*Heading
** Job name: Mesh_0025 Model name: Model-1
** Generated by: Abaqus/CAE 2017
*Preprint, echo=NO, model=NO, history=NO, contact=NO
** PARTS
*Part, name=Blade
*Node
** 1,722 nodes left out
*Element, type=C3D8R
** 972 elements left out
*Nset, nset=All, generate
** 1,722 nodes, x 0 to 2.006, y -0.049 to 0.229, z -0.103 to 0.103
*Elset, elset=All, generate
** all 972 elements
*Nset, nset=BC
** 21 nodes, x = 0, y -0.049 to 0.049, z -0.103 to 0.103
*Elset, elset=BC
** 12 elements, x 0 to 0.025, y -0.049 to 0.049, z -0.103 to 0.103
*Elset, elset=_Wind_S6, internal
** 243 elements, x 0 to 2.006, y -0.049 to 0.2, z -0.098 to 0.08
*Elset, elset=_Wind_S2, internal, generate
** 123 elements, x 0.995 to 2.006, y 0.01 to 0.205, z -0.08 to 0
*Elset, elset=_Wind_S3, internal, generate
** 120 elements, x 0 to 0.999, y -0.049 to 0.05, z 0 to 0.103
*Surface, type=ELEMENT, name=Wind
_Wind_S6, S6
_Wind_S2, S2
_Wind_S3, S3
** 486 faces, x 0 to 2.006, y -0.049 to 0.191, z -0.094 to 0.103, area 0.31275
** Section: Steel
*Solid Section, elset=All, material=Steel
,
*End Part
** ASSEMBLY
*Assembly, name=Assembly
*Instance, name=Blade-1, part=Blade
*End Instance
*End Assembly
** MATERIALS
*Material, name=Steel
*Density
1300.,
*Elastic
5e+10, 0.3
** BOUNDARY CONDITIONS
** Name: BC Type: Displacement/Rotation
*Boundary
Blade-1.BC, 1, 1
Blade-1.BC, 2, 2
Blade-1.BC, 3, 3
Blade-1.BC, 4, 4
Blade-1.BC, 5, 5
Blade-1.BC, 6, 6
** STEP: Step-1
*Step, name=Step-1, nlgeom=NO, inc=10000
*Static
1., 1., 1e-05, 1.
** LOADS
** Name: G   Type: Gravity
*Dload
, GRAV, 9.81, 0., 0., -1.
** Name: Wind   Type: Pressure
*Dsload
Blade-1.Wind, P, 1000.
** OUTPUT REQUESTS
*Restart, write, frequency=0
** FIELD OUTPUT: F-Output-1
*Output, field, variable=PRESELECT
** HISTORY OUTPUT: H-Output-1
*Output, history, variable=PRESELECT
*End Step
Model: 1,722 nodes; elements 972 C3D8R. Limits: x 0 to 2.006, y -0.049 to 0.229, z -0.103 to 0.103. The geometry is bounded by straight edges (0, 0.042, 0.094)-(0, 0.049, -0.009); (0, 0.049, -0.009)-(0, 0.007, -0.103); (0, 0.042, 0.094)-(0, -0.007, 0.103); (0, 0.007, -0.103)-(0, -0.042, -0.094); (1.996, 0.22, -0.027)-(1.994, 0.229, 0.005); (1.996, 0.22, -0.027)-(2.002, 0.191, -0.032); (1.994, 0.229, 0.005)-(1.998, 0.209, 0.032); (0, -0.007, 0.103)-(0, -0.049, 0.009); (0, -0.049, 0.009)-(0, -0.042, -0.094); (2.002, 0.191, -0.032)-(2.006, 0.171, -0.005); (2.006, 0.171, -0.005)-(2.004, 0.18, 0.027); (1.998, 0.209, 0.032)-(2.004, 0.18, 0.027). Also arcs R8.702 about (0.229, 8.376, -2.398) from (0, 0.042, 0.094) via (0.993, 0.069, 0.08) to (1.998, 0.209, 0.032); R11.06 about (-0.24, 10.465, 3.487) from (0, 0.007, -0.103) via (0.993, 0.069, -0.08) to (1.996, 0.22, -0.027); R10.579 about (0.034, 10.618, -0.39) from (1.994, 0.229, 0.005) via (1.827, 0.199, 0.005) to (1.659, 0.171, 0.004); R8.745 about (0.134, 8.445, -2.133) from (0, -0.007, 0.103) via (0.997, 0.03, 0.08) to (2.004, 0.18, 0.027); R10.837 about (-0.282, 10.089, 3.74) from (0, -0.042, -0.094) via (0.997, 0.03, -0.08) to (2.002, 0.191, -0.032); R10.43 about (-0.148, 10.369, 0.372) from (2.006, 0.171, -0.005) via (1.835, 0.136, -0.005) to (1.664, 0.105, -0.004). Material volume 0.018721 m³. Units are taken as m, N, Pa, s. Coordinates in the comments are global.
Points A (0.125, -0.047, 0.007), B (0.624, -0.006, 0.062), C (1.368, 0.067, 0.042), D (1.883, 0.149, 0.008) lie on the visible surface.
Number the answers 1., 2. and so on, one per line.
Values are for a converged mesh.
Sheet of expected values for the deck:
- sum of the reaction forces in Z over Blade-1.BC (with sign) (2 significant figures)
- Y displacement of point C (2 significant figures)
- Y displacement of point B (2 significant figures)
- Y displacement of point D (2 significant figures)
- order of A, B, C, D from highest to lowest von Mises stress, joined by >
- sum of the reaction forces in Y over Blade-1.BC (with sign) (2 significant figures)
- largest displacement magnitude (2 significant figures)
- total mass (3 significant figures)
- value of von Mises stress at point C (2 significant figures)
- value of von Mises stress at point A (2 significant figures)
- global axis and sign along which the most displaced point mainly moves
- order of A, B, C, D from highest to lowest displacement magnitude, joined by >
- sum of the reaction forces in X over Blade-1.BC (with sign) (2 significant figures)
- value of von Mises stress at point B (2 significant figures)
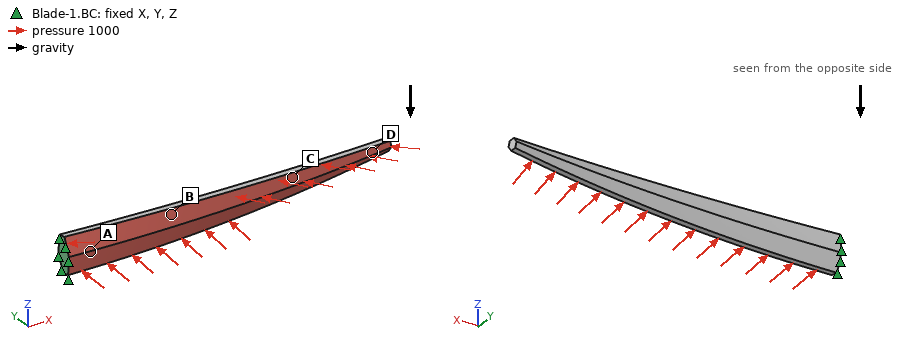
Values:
1. 250 N
2. 4.9e-04 m
3. 1.2e-04 m
4. 8.1e-04 m
5. A > B > C > D
6. -300 N
7. 9.1e-04 m
8. 24.3 kg
9. 2.6e+05 Pa
10. 1.6e+06 Pa
11. +Y
12. D > C > B > A
13. 29 N
14. 8.0e+05 Pa
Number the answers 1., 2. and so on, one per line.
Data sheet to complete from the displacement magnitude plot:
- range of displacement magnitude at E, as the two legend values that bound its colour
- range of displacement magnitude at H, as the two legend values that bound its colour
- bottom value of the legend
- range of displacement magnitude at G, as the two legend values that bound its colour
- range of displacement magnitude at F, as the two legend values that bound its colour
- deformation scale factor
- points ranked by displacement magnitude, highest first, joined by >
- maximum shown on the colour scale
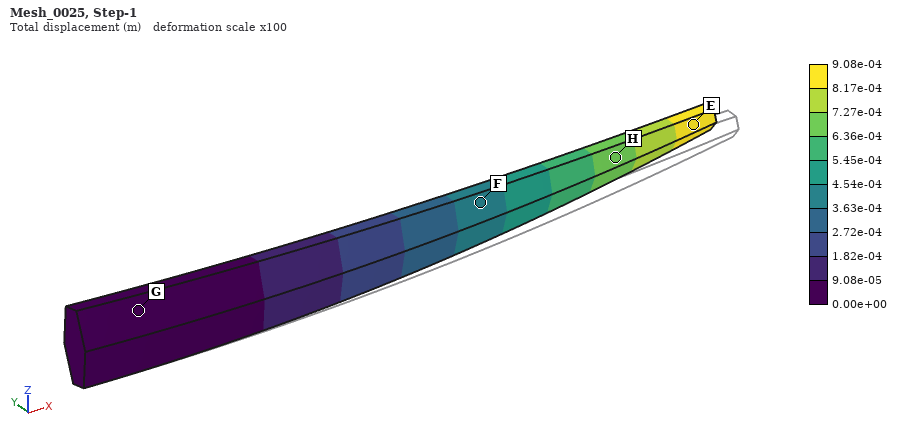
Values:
1. 8.17e-04 to 9.08e-04 m
2. 6.36e-04 to 7.27e-04 m
3. 0.00e+00 m
4. 0.00e+00 to 9.08e-05 m
5. 3.63e-04 to 4.54e-04 m
6. 100
7. E > H > F > G
8. 9.08e-04 m
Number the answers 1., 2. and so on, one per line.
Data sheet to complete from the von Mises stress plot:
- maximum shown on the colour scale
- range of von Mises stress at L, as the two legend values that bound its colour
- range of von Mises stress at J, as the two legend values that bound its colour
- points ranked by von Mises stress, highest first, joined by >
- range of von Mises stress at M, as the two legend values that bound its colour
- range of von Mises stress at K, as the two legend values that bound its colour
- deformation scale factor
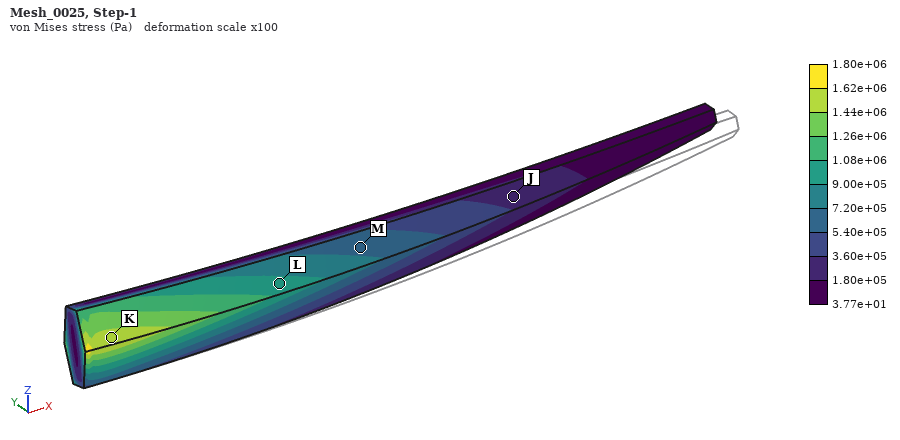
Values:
1. 1.80e+06 Pa
2. 9.00e+05 to 1.08e+06 Pa
3. 1.80e+05 to 3.60e+05 Pa
4. K > L > M > J
5. 5.40e+05 to 7.20e+05 Pa
6. 1.44e+06 to 1.62e+06 Pa
7. 100
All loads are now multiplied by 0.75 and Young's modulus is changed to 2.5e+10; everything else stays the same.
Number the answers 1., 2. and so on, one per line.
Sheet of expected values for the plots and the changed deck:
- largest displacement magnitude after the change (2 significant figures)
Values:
1. 0.0014 m
